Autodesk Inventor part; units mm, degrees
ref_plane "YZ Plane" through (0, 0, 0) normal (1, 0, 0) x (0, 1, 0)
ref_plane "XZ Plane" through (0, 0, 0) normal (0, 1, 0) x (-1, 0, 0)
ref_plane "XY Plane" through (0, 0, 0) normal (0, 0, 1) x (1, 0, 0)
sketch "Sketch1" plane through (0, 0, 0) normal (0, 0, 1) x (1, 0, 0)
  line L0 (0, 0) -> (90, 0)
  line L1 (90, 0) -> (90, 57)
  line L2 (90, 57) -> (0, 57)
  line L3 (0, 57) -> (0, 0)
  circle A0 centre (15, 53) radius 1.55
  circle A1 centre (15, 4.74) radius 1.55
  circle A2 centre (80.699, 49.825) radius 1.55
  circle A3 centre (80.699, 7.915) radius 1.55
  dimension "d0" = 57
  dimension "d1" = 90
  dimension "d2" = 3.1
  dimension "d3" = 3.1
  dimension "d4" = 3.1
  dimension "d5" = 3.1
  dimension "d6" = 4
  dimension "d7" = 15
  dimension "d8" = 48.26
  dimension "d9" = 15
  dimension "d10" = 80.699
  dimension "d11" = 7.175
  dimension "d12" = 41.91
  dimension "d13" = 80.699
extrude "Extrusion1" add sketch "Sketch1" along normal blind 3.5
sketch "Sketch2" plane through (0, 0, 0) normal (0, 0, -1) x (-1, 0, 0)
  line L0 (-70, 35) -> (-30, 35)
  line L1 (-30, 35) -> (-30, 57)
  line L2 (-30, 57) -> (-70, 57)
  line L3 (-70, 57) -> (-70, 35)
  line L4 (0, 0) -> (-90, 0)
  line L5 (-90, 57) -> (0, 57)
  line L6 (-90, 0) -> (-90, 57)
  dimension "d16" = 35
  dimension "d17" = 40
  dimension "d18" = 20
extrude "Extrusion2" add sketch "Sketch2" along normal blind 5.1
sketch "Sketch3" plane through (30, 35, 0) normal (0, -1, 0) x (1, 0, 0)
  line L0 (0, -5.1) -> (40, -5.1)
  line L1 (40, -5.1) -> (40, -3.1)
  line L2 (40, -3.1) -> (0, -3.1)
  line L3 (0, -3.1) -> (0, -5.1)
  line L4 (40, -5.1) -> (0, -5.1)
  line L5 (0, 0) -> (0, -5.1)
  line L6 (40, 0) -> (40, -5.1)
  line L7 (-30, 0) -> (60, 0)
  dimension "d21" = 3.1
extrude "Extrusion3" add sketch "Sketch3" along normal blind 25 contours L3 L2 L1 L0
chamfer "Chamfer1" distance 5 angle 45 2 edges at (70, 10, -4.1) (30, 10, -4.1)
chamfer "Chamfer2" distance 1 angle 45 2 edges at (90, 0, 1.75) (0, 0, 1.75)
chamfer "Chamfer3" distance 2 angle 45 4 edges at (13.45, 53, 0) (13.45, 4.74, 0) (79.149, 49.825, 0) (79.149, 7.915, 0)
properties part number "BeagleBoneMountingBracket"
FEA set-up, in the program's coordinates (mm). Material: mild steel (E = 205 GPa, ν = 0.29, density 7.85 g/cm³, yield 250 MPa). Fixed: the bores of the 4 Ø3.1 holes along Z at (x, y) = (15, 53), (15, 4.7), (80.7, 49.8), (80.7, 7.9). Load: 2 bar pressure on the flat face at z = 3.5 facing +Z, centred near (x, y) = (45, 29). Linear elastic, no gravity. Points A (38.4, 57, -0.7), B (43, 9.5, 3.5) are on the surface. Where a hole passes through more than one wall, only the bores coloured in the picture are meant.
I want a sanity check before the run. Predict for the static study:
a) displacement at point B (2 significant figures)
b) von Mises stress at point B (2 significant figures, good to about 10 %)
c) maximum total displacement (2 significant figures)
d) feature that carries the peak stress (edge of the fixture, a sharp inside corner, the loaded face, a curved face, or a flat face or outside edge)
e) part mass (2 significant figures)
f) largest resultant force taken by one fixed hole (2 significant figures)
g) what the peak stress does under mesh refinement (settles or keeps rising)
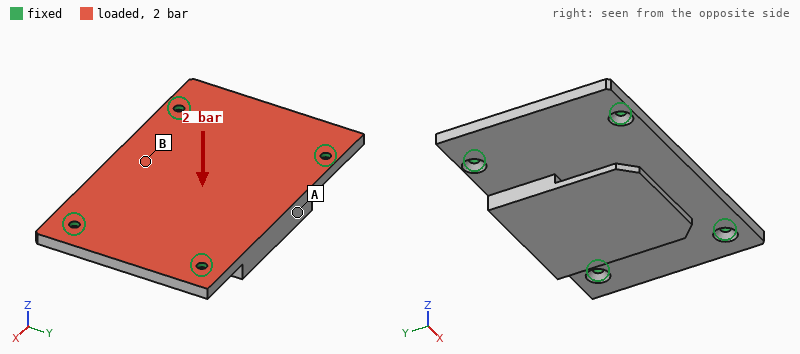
19 µm
16 MPa
27 µm
edge of the fixture
190 g
450 N
keeps rising
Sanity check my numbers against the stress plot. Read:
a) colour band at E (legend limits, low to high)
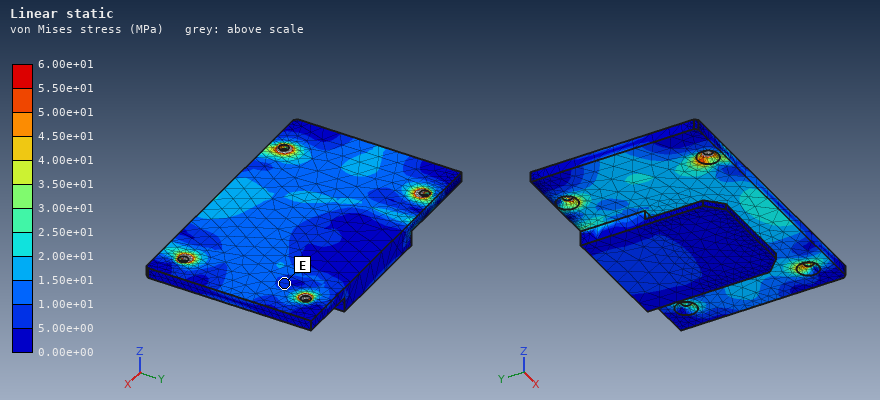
5.00e+00 to 1.00e+01 MPa
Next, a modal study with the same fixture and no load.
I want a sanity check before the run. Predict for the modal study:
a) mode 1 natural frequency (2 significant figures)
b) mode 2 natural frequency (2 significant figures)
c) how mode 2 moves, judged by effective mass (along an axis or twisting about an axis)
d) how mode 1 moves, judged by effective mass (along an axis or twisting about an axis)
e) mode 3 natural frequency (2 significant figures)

2200 Hz
3600 Hz
along Z
along Z
4600 Hz
